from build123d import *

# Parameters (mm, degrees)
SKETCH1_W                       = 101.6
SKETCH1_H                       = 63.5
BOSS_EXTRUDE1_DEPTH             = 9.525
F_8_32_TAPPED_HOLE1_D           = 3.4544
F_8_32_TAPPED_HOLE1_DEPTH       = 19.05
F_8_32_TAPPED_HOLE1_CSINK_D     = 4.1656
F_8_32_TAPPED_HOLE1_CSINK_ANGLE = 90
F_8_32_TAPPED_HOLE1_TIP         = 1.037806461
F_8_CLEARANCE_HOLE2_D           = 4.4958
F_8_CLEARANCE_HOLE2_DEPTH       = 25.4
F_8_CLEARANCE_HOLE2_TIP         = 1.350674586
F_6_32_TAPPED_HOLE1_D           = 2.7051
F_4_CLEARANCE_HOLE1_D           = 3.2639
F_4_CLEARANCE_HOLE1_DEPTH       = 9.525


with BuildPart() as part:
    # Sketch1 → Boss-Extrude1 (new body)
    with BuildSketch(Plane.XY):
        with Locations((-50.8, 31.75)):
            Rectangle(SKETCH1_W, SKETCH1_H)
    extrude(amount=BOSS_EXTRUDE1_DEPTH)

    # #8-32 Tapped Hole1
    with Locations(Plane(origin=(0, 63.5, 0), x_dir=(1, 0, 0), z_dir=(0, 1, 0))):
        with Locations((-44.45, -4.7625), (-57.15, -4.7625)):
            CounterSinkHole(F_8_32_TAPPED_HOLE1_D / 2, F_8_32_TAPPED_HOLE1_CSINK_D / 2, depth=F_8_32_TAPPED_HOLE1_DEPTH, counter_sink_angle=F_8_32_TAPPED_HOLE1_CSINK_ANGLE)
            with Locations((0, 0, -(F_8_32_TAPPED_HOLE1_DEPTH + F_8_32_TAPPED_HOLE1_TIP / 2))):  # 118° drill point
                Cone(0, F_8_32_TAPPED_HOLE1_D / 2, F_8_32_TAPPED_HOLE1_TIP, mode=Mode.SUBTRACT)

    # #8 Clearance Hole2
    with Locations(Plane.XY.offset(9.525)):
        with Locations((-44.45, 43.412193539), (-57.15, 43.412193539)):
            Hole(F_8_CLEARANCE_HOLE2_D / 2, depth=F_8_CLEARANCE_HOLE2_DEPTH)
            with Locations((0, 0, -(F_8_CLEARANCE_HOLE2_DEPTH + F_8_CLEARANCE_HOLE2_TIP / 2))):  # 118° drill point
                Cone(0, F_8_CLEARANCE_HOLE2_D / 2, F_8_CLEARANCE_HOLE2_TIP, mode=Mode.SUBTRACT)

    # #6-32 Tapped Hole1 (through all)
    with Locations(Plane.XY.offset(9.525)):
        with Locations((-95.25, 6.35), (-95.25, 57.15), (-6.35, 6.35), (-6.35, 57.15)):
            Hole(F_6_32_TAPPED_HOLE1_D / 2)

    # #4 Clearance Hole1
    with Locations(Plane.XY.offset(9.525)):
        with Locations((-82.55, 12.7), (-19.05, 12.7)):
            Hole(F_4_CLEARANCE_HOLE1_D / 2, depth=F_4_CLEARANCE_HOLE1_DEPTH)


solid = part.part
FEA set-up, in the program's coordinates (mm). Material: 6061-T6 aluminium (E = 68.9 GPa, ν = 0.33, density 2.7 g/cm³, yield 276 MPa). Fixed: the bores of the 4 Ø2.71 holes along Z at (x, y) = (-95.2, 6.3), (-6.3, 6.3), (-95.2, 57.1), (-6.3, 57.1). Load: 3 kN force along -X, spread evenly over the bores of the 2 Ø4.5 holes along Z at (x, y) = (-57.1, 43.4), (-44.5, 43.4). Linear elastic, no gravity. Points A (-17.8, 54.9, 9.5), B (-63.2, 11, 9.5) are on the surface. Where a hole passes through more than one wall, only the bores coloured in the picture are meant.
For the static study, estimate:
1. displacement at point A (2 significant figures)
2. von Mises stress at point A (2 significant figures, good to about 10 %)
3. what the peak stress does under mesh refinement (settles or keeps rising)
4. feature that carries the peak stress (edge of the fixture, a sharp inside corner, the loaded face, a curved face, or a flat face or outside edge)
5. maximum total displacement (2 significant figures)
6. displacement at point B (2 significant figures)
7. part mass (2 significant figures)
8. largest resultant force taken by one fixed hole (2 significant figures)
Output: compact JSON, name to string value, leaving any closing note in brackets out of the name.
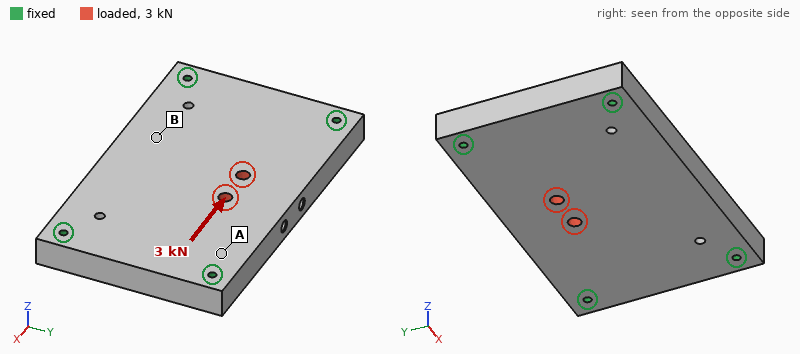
{"displacement at point A": "1.4 µm", "von Mises stress at point A": "5.8 MPa", "what the peak stress does under mesh refinement": "keeps rising", "feature that carries the peak stress": "a sharp inside corner", "maximum total displacement": "4.9 µm", "displacement at point B": "1.3 µm", "part mass": "160 g", "largest resultant force taken by one fixed hole": "930 N"}
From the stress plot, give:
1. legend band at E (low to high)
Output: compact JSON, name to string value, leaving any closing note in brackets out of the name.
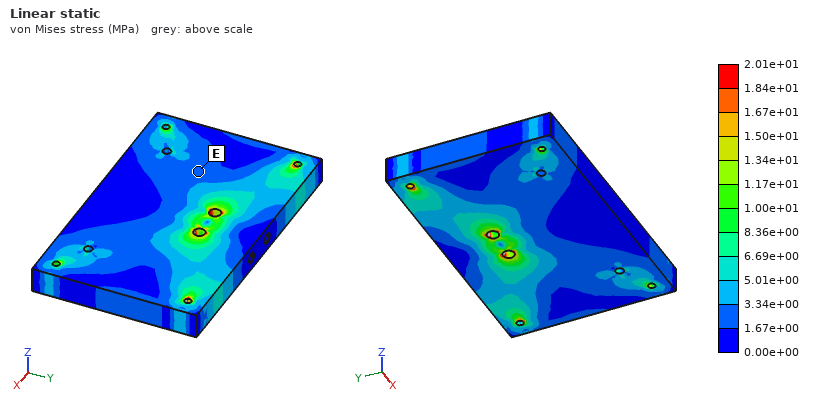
{"legend band at E": "1.67e+00 to 3.34e+00 MPa"}
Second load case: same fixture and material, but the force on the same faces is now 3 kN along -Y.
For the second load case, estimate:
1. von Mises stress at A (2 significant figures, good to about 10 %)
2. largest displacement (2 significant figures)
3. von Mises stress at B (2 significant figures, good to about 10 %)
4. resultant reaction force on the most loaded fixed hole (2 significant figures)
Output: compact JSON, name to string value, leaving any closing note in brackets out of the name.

{"von Mises stress at A": "4.4 MPa", "largest displacement": "7.4 µm", "von Mises stress at B": "3.2 MPa", "resultant reaction force on the most loaded fixed hole": "980 N"}
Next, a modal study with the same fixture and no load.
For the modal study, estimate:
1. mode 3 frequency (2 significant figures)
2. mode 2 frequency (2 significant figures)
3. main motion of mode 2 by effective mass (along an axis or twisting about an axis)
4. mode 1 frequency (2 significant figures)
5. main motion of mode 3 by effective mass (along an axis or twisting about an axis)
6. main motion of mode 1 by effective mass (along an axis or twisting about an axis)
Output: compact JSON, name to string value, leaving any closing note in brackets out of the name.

{"mode 3 frequency": "11 kHz", "mode 2 frequency": "7200 Hz", "main motion of mode 2 by effective mass": "twisting about X", "mode 1 frequency": "4500 Hz", "main motion of mode 3 by effective mass": "twisting about Y", "main motion of mode 1 by effective mass": "along Z"}
